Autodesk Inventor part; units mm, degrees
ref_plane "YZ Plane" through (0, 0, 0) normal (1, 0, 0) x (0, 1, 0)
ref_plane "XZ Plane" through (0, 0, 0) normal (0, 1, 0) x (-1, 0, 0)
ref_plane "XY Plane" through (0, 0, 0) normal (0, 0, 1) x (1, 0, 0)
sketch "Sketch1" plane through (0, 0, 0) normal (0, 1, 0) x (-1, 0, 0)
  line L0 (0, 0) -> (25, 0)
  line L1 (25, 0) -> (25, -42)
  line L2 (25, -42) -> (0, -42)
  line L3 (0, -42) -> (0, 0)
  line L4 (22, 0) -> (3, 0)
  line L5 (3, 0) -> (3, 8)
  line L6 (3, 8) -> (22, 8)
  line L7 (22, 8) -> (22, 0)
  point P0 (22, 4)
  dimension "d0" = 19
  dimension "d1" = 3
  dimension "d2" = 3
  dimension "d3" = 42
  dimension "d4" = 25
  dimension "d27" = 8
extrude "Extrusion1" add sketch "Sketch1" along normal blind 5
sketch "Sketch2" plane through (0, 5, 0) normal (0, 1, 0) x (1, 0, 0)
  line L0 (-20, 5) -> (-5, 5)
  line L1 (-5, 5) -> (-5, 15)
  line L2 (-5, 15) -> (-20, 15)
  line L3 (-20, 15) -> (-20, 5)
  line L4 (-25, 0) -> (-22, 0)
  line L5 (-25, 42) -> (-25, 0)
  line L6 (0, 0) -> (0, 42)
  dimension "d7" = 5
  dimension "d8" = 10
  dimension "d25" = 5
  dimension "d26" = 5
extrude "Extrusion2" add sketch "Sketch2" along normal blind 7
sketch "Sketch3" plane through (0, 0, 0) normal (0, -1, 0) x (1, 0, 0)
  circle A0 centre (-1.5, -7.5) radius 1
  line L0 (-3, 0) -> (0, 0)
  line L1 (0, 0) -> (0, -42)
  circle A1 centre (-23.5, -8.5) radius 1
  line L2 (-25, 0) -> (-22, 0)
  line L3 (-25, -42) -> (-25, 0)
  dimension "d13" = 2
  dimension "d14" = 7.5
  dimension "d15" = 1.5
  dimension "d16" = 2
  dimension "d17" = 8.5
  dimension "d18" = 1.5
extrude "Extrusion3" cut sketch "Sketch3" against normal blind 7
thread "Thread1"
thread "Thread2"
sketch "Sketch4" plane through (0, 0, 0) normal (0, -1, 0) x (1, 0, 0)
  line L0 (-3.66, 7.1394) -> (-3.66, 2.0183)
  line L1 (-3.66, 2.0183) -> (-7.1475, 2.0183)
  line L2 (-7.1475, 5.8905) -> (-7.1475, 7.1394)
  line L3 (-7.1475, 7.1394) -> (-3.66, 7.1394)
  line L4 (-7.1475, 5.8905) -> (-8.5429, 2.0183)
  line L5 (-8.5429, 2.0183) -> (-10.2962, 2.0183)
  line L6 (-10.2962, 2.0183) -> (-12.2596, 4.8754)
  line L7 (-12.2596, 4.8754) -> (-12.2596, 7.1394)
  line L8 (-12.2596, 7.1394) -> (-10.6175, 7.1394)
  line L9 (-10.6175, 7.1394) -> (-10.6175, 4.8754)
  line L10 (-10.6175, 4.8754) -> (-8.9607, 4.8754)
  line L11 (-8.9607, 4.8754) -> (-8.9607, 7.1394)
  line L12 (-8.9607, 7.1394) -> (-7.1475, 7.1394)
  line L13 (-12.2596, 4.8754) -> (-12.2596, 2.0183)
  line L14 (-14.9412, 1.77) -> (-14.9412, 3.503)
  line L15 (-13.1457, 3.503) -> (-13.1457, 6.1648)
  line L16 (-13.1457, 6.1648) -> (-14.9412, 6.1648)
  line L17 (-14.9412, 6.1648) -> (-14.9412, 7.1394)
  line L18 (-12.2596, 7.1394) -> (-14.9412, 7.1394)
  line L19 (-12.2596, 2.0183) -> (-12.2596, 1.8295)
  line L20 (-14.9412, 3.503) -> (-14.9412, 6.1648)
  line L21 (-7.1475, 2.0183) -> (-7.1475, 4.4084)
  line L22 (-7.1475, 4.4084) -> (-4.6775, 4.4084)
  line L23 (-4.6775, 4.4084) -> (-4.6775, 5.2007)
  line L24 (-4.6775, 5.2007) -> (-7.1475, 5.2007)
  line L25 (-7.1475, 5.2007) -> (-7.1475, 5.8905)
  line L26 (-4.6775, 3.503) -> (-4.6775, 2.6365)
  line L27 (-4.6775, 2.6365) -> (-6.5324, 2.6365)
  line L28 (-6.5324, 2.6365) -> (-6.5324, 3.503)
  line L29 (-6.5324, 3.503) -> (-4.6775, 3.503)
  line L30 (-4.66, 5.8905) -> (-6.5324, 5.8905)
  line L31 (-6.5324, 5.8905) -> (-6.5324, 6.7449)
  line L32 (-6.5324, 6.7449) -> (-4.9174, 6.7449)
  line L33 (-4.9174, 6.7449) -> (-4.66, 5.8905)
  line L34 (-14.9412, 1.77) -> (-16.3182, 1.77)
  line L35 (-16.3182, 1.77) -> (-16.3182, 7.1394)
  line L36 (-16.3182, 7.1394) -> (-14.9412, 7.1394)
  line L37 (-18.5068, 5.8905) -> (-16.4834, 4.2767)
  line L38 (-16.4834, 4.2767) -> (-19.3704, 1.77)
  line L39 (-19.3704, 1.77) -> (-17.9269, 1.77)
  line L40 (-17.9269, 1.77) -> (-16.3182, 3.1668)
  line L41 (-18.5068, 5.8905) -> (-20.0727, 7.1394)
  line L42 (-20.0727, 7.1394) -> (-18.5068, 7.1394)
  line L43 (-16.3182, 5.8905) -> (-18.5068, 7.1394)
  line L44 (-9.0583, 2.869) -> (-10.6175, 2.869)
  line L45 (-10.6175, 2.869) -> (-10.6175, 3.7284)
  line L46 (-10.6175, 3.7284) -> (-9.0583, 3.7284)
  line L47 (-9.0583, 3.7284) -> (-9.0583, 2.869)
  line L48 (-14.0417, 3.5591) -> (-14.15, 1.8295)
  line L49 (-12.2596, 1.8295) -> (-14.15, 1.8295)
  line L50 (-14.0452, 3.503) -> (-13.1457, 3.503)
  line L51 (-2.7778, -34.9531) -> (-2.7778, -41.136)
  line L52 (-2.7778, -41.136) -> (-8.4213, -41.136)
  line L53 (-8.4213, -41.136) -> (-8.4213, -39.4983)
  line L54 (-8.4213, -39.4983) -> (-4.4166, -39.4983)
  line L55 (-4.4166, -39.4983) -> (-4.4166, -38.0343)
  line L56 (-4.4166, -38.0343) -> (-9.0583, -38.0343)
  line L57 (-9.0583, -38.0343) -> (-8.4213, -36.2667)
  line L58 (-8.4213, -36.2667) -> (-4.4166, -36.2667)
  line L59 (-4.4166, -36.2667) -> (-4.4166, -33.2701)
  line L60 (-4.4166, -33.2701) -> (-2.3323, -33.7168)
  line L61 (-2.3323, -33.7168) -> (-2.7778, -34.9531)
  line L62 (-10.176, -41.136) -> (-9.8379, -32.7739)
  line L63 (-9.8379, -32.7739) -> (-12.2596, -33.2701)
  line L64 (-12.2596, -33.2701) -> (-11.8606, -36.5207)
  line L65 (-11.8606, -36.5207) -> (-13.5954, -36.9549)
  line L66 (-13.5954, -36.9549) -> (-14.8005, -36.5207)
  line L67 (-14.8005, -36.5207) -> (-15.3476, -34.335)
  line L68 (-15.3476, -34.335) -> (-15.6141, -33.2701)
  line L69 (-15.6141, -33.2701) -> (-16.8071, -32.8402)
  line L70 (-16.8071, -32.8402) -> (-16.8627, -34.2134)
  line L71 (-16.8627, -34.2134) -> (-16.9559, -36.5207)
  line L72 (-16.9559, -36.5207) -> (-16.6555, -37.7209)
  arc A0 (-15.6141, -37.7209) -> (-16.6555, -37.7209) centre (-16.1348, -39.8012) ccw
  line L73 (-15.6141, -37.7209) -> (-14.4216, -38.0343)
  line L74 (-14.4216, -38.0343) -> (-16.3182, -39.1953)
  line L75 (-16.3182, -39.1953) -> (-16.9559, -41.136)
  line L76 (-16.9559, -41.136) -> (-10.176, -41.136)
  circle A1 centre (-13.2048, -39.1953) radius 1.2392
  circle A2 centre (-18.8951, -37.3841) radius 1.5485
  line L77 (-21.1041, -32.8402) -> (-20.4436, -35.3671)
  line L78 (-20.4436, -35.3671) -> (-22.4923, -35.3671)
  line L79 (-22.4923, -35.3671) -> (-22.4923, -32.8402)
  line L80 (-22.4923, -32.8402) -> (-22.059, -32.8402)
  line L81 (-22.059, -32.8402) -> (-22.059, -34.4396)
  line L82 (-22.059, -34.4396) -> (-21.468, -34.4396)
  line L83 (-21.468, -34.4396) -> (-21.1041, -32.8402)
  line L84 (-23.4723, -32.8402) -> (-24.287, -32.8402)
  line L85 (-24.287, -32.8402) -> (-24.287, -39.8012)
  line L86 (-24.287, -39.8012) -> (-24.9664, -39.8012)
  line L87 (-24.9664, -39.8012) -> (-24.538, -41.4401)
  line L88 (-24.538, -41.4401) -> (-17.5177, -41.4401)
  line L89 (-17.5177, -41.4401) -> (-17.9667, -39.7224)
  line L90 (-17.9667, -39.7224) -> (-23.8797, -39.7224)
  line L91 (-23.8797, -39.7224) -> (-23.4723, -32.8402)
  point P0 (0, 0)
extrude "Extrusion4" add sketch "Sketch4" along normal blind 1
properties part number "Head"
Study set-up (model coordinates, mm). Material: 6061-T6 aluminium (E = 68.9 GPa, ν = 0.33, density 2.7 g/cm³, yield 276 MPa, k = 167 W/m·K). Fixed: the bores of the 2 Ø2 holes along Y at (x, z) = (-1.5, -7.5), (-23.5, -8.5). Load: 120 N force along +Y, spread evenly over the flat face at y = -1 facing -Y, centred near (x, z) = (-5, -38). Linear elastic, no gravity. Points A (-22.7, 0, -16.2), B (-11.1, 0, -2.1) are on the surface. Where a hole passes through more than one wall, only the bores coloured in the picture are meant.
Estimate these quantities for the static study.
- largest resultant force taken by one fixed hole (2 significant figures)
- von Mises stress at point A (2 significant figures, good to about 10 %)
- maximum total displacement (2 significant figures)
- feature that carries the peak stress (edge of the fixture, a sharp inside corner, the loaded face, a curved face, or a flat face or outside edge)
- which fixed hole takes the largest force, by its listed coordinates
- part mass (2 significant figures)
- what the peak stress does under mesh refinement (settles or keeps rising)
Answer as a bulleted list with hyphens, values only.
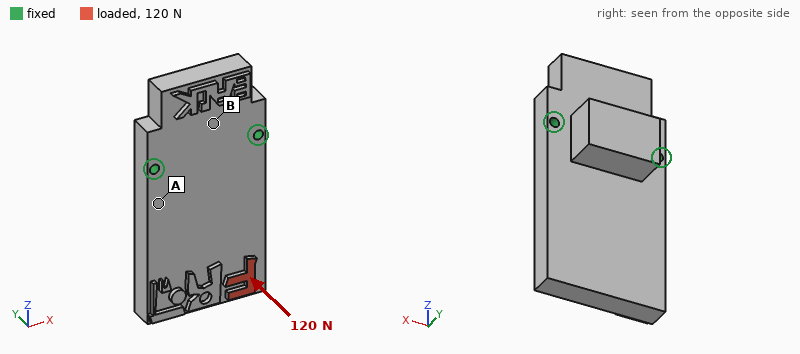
- 100 N
- 22 MPa
- 92 µm
- edge of the fixture
- (-1.5, -7.5)
- 19 g
- keeps rising
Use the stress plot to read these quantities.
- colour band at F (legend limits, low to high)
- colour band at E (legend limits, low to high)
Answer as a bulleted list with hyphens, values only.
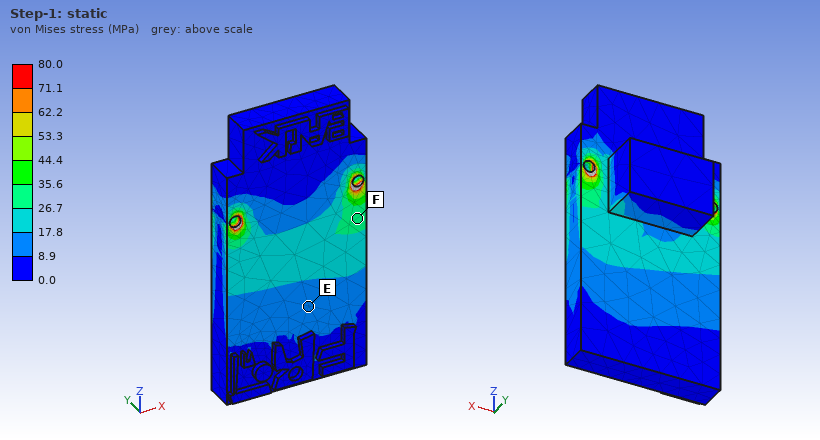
- 26.7 to 35.6 MPa
- 8.9 to 17.8 MPa
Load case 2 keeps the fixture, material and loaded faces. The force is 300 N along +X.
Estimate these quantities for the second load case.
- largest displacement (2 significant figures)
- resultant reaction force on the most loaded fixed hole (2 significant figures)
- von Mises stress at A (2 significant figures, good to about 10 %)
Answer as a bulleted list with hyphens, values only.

- 20 µm
- 440 N
- 10 MPa
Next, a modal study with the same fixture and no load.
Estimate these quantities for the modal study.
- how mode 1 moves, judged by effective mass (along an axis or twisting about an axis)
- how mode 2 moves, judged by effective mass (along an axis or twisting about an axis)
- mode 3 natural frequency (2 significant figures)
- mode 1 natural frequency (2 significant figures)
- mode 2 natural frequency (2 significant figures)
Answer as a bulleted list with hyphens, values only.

- along Y
- twisting about Z
- 13 kHz
- 3100 Hz
- 10 kHz
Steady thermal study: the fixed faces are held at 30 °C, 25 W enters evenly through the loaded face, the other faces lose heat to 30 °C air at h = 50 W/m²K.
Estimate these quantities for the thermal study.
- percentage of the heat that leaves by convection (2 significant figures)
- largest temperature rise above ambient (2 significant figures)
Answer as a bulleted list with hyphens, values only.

- 11 %
- 54 K
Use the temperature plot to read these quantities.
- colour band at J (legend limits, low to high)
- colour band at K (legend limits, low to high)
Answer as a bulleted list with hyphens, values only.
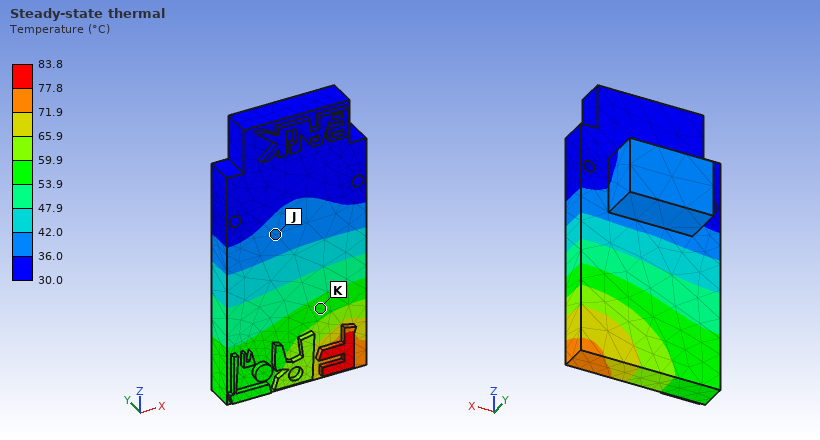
- 36.0 to 42.0 °C
- 53.9 to 59.9 °C
